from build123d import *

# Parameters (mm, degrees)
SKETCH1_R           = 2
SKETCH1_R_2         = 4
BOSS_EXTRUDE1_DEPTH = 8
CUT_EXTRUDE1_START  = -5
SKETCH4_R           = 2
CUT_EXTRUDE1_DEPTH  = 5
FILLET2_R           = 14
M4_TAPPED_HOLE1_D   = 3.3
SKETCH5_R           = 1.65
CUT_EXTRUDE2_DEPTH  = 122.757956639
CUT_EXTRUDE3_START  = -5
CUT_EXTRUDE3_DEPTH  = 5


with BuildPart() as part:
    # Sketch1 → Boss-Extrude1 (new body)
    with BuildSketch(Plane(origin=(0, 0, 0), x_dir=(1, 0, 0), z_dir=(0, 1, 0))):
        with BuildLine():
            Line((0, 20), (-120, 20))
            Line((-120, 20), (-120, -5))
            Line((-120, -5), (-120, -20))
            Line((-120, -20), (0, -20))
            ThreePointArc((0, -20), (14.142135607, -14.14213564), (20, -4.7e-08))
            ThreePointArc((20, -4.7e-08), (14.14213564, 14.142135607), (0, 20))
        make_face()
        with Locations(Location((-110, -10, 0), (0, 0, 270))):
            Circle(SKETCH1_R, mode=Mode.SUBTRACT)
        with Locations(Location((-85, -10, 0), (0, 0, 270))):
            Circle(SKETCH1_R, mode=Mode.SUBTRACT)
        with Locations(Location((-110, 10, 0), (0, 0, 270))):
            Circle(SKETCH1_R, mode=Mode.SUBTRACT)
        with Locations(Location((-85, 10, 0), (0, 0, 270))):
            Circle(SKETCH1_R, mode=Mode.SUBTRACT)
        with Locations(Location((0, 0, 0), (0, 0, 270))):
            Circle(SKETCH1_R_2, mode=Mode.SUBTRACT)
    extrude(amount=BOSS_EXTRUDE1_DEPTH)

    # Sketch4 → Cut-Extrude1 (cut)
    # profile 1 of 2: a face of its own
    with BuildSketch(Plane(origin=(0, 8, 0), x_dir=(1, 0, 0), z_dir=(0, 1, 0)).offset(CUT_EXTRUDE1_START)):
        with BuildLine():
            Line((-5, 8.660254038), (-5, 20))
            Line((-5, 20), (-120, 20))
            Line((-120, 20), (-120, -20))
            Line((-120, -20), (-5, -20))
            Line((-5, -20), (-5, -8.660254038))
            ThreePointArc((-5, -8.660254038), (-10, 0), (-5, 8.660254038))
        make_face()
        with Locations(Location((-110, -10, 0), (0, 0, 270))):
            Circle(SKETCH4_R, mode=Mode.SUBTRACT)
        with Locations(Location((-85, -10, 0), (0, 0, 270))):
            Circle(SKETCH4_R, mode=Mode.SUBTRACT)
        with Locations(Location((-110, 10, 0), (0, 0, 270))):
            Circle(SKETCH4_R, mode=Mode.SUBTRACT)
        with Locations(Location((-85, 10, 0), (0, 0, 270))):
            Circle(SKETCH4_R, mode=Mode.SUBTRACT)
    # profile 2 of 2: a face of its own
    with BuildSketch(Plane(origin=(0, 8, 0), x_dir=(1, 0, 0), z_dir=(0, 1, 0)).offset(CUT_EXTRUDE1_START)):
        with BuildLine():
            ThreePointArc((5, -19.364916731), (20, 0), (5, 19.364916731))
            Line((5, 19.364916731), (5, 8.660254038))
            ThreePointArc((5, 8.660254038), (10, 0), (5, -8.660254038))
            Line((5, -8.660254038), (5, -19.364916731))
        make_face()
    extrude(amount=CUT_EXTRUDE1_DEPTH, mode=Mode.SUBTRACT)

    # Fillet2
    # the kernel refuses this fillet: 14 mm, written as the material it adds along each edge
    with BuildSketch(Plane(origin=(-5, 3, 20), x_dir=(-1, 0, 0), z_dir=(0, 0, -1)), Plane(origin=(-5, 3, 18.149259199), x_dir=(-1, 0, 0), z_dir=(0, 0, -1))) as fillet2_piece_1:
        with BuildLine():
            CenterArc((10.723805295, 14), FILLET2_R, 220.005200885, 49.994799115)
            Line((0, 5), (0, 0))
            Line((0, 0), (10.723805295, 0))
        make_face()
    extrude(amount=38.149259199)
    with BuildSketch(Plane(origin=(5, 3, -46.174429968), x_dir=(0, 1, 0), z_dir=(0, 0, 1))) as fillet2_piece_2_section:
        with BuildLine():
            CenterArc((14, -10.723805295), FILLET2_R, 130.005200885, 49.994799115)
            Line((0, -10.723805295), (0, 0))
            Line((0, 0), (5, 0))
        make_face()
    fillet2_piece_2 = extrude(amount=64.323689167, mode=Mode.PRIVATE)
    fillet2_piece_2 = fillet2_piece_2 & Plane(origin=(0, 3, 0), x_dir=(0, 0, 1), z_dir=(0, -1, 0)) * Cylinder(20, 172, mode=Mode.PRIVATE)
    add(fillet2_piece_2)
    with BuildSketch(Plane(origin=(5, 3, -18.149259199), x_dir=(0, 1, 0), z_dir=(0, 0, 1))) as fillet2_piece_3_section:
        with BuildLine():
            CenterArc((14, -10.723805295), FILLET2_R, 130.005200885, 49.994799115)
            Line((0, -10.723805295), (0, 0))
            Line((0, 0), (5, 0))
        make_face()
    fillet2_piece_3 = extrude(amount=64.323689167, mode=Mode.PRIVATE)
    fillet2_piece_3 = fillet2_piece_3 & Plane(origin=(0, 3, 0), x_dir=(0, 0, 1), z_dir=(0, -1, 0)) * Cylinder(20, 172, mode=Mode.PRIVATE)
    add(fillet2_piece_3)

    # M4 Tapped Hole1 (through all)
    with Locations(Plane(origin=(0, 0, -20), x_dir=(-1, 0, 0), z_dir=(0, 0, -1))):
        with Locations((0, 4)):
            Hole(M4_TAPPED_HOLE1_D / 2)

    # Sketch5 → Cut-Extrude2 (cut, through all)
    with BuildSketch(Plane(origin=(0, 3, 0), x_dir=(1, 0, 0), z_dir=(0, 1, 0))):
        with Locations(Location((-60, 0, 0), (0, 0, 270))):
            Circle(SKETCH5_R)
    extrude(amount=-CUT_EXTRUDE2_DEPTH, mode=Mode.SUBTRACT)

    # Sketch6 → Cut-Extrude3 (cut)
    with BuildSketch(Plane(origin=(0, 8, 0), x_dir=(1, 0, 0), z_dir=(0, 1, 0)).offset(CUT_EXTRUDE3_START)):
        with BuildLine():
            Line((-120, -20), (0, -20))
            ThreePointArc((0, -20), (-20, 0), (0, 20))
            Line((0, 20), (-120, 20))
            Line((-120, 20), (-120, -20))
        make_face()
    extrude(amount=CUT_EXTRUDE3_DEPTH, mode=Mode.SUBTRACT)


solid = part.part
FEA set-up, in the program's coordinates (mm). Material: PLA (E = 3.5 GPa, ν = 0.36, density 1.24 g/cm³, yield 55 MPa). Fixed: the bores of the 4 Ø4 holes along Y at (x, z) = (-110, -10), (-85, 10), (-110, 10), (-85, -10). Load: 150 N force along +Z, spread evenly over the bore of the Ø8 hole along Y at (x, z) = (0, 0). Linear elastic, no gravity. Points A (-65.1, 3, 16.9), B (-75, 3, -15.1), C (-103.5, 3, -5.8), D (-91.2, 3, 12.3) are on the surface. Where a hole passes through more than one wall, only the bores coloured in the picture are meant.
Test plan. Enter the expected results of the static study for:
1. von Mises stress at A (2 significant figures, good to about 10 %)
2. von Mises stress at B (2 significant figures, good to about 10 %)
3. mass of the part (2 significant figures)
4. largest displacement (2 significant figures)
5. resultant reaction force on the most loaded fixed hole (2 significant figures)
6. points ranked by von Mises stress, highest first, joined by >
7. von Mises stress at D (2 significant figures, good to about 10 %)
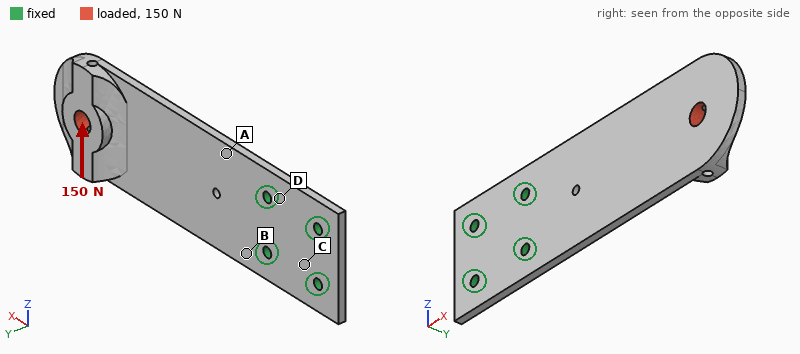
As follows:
11 MPa
8.8 MPa
23 g
1.5 mm
430 N
A > B > D > C
3.7 MPa
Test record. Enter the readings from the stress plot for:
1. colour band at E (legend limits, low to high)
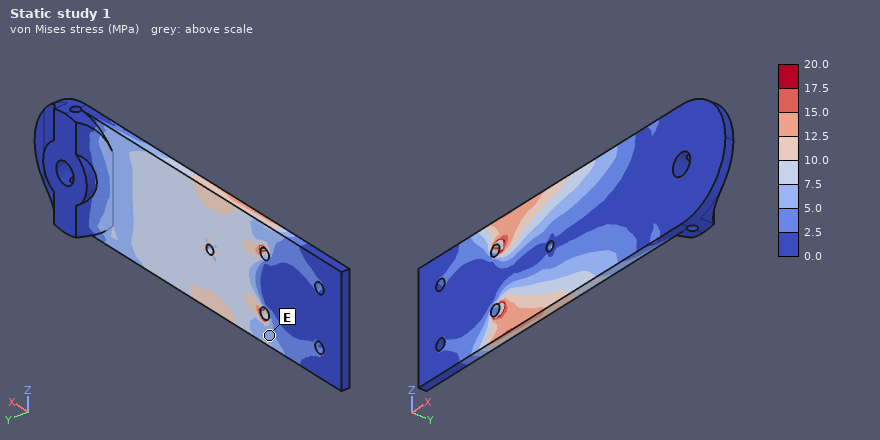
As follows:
5.0 to 7.5 MPa
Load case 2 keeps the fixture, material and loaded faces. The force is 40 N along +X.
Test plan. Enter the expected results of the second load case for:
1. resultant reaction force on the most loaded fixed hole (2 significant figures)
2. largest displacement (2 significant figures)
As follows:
17 N
1.5 mm
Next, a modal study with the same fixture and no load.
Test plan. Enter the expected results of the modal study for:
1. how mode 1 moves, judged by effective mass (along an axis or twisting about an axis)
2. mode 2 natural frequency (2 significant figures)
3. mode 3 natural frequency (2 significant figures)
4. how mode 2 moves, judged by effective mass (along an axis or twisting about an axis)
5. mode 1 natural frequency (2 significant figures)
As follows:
along Y
360 Hz
500 Hz
twisting about X
65 Hz
